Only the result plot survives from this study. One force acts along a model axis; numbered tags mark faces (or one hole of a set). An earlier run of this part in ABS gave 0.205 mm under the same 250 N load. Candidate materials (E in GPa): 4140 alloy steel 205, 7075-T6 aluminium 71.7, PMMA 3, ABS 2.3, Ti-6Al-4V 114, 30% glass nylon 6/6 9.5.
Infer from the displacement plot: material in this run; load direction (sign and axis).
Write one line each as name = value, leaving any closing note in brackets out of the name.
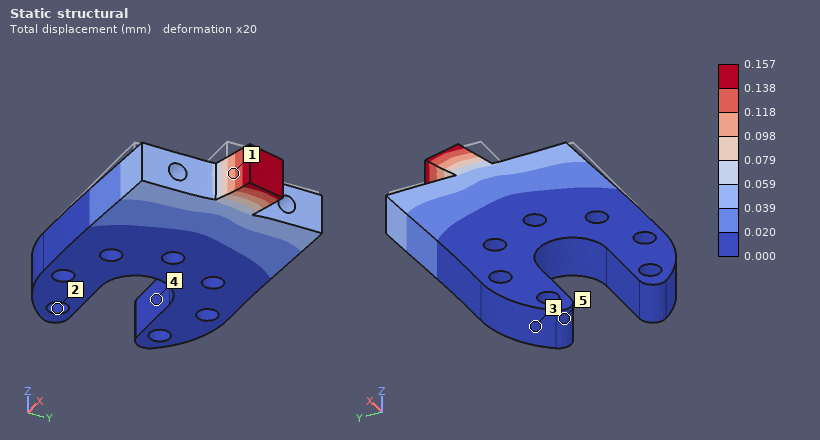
material in this run = PMMA
load direction = +Y
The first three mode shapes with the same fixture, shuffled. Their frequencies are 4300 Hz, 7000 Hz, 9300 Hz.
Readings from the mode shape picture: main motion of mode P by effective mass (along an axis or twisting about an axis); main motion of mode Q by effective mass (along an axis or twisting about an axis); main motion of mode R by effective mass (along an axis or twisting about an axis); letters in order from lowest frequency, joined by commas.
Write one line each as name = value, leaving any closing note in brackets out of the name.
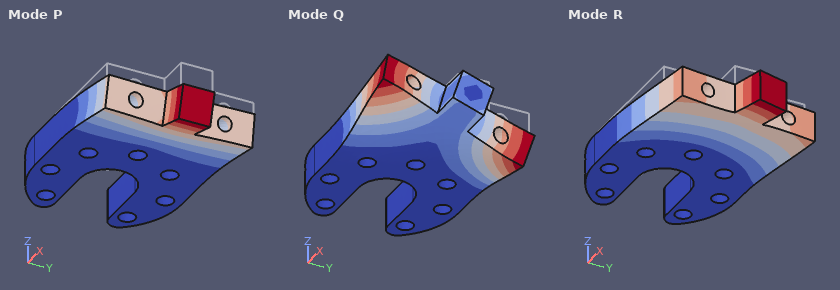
main motion of mode P by effective mass = along Z
main motion of mode Q by effective mass = twisting about X
main motion of mode R by effective mass = along Y
letters in order from lowest frequency, joined by commas = P, Q, R
